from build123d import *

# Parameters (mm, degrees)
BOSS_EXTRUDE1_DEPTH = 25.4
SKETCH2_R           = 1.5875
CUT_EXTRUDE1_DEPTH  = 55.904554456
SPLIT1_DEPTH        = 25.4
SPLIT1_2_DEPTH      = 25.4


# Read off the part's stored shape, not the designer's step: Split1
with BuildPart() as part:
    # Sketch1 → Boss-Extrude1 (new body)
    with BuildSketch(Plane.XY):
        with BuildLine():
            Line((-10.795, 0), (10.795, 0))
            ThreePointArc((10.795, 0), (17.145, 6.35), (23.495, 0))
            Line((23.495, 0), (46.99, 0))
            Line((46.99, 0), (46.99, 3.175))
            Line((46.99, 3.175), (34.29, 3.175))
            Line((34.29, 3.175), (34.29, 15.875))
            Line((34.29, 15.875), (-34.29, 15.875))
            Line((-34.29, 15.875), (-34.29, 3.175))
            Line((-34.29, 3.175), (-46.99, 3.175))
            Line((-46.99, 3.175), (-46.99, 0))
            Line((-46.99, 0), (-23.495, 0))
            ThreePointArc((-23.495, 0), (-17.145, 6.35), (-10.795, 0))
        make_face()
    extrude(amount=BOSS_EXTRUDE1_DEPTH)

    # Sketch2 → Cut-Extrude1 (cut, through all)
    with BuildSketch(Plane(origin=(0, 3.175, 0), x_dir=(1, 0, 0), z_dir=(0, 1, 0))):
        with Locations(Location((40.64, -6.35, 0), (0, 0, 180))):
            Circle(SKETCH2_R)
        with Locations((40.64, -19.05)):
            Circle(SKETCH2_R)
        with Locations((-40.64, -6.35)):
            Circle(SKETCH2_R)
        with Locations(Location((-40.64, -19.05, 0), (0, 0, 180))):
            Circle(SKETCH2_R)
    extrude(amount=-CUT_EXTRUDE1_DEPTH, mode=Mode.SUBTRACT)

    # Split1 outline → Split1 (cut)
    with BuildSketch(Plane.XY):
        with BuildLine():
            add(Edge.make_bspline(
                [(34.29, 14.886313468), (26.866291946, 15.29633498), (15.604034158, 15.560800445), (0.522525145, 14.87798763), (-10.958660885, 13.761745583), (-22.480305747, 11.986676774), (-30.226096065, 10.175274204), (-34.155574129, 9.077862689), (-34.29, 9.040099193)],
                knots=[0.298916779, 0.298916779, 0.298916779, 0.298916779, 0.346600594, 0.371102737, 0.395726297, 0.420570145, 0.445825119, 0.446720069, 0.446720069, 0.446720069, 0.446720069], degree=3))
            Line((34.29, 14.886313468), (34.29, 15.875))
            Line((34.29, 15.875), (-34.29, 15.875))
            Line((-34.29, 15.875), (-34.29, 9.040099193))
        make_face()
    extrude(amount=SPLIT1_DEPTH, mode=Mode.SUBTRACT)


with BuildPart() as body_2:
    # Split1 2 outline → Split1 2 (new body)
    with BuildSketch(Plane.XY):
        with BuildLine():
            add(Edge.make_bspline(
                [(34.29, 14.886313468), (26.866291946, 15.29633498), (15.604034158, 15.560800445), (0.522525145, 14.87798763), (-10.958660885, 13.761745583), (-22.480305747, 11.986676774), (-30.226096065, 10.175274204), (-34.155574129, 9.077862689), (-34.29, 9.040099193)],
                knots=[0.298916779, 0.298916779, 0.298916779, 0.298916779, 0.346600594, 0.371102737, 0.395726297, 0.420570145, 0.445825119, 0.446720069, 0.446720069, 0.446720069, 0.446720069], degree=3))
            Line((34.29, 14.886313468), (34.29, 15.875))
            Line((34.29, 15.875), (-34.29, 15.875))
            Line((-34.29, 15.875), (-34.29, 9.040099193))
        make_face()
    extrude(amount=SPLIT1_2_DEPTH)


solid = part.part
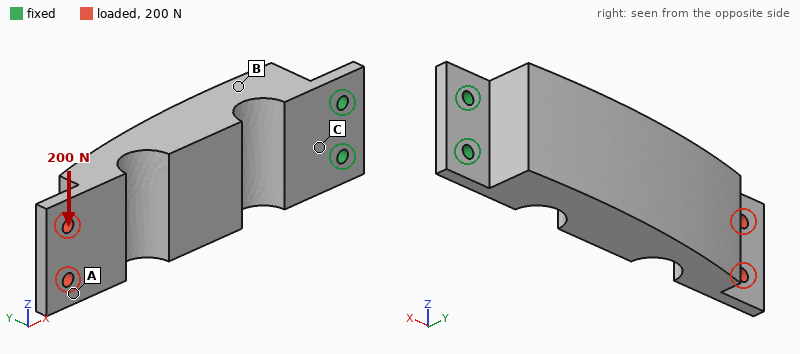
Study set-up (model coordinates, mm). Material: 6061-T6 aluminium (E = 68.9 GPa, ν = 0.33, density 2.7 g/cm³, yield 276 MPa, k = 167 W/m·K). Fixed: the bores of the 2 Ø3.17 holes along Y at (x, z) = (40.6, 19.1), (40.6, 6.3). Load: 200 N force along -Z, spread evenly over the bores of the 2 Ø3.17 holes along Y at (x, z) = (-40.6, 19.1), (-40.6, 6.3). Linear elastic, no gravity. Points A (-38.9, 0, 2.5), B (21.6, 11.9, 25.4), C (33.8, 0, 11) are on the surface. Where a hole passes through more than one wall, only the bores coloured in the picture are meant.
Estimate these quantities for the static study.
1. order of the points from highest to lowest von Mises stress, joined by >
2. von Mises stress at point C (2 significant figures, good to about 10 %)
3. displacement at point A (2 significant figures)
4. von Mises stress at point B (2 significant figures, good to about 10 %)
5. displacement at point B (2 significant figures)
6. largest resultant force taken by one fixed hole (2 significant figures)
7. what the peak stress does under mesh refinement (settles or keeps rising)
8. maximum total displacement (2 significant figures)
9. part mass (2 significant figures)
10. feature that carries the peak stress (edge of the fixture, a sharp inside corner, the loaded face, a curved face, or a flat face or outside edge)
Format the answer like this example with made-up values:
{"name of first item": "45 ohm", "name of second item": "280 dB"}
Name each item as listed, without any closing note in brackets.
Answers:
{"order of the points from highest to lowest von Mises stress, joined by >": "C > B > A", "von Mises stress at point C": "25 MPa", "displacement at point A": "0.11 mm", "von Mises stress at point B": "11 MPa", "displacement at point B": "0.020 mm", "largest resultant force taken by one fixed hole": "1.1 kN", "what the peak stress does under mesh refinement": "keeps rising", "maximum total displacement": "0.12 mm", "part mass": "62 g", "feature that carries the peak stress": "edge of the fixture"}
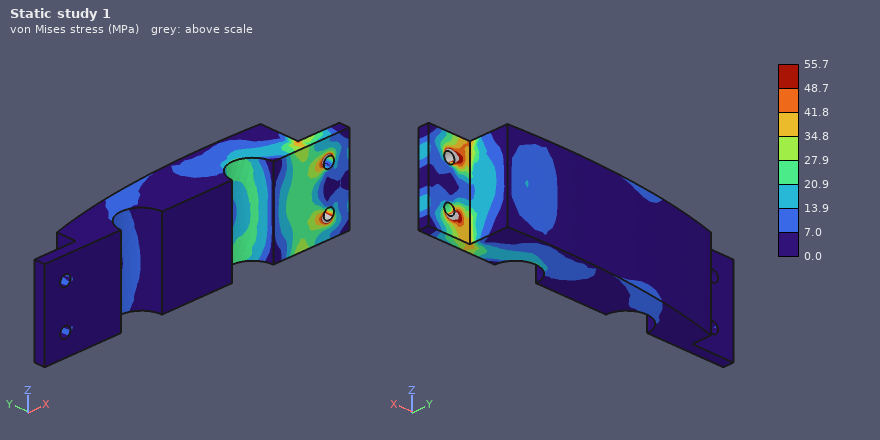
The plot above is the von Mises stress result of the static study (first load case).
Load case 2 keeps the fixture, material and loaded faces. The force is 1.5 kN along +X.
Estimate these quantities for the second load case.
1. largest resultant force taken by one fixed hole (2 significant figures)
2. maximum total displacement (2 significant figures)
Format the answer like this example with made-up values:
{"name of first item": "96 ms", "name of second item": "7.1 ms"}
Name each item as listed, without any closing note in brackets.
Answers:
{"largest resultant force taken by one fixed hole": "750 N", "maximum total displacement": "0.26 mm"}
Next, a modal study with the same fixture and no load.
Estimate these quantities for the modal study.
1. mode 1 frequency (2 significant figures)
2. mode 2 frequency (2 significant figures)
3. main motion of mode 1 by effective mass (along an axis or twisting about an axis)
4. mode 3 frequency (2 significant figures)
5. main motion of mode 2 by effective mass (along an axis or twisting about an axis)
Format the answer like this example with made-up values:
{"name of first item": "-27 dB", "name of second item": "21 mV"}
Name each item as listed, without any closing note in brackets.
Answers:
{"mode 1 frequency": "380 Hz", "mode 2 frequency": "1800 Hz", "main motion of mode 1 by effective mass": "along Y", "mode 3 frequency": "3900 Hz", "main motion of mode 2 by effective mass": "along Z"}
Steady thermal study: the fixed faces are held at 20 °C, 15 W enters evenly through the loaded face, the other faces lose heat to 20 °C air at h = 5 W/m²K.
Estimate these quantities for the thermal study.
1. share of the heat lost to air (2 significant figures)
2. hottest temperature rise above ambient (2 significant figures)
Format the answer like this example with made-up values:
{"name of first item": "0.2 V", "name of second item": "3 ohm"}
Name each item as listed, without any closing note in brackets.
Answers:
{"share of the heat lost to air": "5.0 %", "hottest temperature rise above ambient": "44 K"}
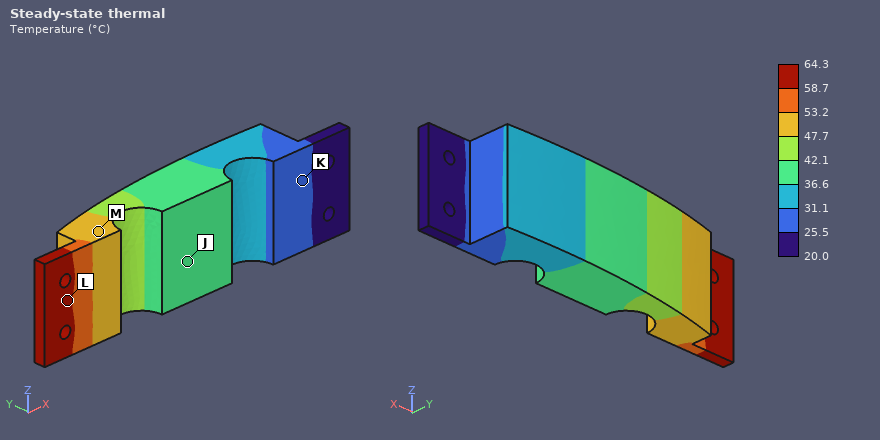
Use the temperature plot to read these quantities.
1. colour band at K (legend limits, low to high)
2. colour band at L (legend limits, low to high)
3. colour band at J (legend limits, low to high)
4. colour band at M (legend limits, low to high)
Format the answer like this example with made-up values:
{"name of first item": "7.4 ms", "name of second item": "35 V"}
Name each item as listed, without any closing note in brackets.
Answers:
{"colour band at K": "25.5 to 31.1 °C", "colour band at L": "58.7 to 64.3 °C", "colour band at J": "36.6 to 42.1 °C", "colour band at M": "47.7 to 53.2 °C"}
